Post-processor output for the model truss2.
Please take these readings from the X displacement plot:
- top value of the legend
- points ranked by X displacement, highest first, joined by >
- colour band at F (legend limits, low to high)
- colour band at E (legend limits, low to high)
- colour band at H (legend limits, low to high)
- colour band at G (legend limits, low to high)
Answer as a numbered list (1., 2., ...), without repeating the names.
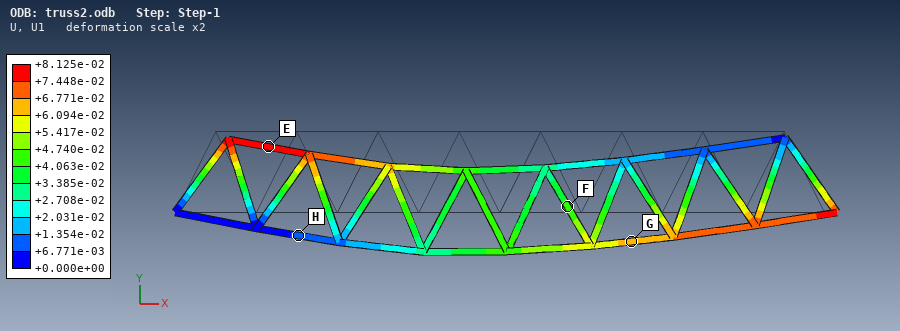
1. +8.125e-02
2. E > G > F > H
3. +4.063e-02 to +4.740e-02
4. +7.448e-02 to +8.125e-02
5. +6.771e-03 to +1.354e-02
6. +6.094e-02 to +6.771e-02
